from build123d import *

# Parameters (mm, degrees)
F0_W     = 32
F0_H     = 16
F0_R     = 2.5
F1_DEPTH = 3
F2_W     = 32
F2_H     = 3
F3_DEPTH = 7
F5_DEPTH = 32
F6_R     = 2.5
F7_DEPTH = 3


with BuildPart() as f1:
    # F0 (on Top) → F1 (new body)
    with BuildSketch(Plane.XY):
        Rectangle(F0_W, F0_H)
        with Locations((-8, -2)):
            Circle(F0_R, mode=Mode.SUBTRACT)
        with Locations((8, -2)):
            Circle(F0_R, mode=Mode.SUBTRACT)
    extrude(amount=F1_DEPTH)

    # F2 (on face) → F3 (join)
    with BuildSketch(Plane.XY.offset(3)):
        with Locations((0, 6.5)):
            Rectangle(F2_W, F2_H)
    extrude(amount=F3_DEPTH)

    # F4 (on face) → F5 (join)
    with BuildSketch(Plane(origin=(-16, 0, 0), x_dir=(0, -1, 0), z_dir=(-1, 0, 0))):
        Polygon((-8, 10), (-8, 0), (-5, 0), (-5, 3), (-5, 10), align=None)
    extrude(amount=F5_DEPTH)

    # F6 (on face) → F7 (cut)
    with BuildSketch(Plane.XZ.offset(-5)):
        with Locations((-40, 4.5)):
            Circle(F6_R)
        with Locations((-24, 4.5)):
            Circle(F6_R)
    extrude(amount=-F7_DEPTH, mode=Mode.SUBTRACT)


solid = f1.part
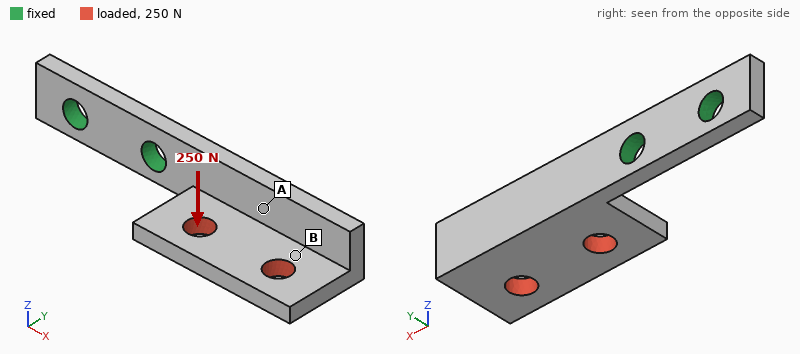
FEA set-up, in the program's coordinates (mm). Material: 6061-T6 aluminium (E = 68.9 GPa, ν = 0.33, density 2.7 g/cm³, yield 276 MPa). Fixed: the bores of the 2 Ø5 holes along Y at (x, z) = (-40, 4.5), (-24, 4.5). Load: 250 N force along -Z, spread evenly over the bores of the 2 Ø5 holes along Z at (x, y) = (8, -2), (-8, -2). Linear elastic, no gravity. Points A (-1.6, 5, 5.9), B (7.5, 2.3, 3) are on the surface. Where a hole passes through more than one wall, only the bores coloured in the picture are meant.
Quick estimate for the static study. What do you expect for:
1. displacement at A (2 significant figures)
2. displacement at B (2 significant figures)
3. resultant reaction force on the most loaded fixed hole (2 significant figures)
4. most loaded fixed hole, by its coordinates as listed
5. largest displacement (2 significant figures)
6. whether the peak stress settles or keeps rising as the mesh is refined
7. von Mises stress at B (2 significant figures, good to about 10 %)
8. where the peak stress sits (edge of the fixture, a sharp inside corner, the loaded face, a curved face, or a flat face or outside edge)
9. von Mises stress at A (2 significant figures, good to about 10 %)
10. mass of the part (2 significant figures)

0.087 mm
0.18 mm
320 N
(-24, 4.5)
0.40 mm
keeps rising
21 MPa
edge of the fixture
55 MPa
7.9 g
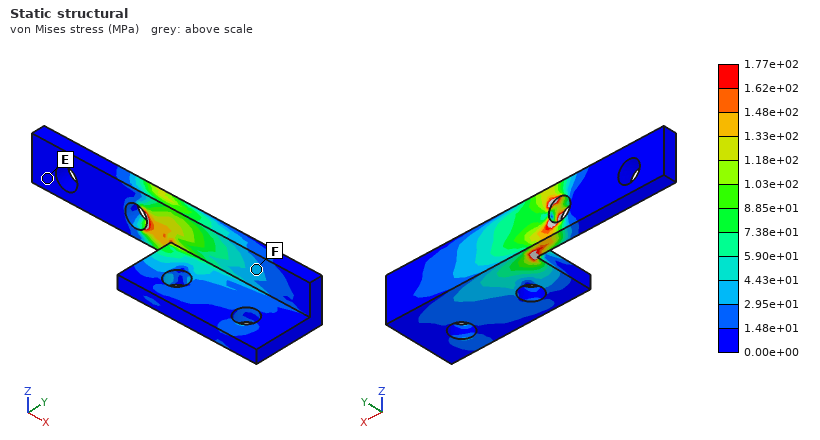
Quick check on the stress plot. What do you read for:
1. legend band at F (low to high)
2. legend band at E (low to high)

2.95e+01 to 4.43e+01 MPa
0.00e+00 to 1.48e+01 MPa
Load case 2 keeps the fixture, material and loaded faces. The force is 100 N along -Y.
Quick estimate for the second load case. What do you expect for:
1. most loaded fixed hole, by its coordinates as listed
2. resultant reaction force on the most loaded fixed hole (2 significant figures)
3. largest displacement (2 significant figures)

(-24, 4.5)
100 N
0.41 mm
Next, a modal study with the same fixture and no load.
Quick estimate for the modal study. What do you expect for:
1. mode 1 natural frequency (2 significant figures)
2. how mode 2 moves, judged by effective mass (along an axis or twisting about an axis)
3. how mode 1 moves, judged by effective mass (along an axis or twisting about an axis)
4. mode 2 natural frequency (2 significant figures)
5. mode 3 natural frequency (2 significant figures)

1300 Hz
along Z
along Y
2800 Hz
5200 Hz
